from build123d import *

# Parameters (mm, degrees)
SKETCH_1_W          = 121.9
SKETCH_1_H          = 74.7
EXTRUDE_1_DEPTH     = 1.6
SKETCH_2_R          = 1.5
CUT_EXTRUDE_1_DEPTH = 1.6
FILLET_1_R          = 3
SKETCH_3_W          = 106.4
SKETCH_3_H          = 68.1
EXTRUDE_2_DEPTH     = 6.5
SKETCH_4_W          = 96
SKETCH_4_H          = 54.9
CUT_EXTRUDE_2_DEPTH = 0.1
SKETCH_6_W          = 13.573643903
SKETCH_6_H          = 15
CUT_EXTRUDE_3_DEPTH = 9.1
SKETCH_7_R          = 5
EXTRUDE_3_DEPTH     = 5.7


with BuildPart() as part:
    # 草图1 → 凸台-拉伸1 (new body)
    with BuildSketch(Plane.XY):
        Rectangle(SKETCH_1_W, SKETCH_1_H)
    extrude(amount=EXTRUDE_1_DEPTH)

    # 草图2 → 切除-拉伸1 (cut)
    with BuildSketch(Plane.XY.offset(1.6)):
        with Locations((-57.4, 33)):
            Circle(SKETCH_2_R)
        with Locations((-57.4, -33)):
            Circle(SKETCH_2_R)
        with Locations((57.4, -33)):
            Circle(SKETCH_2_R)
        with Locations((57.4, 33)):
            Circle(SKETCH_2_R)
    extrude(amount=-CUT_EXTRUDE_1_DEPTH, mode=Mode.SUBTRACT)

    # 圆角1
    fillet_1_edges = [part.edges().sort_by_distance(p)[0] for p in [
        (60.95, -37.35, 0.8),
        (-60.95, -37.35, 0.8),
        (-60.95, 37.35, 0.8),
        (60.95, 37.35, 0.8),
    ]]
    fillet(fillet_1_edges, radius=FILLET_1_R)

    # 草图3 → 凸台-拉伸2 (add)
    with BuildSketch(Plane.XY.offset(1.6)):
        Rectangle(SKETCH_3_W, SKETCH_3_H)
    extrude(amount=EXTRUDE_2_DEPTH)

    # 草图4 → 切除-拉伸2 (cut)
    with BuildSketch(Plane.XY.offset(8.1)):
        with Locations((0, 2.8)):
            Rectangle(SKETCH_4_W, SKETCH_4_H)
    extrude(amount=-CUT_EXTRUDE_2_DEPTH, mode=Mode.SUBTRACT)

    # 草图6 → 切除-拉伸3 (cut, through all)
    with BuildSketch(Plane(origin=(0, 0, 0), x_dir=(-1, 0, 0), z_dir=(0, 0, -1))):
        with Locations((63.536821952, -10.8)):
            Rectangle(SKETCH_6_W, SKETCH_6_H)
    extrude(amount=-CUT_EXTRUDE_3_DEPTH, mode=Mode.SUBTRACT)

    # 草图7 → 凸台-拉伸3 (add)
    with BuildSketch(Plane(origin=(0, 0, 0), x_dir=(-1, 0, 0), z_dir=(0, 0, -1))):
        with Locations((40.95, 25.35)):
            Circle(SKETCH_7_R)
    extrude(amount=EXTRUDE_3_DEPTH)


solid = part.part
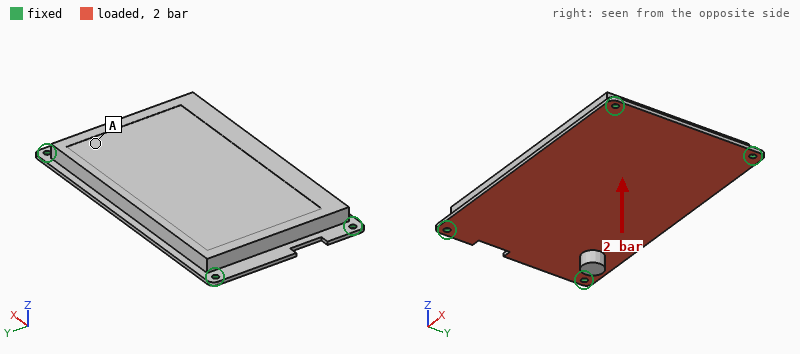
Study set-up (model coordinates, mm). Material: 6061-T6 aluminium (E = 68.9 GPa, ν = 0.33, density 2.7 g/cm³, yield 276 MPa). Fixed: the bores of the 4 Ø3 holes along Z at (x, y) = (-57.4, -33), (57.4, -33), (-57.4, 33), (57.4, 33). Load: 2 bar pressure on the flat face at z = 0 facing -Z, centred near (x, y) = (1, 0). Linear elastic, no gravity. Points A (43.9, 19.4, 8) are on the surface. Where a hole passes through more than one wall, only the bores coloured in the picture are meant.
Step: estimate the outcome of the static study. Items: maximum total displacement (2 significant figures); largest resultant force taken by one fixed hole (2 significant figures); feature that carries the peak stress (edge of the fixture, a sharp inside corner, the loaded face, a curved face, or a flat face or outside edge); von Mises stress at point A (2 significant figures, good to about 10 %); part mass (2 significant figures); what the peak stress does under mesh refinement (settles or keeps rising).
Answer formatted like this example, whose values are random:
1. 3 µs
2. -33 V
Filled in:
1. 0.12 mm
2. 1.0 kN
3. edge of the fixture
4. 15 MPa
5. 170 g
6. keeps rising
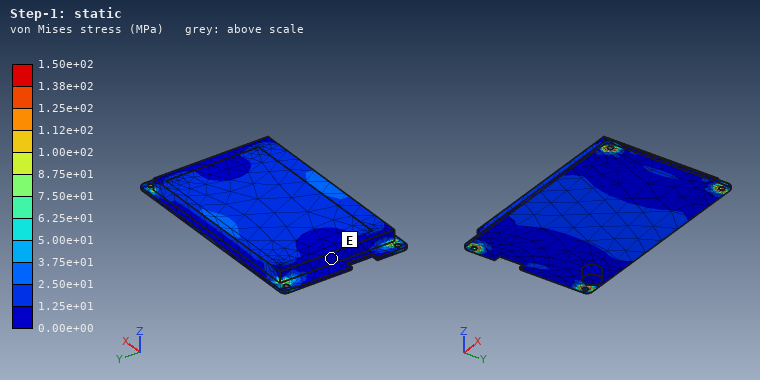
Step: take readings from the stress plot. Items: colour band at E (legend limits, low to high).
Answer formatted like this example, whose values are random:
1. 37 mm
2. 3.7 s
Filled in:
1. 0.00e+00 to 1.25e+01 MPa
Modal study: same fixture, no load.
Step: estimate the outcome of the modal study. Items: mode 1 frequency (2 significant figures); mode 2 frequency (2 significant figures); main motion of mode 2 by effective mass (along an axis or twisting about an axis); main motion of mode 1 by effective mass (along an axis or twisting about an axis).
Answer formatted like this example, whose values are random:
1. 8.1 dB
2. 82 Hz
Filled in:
1. 1600 Hz
2. 3100 Hz
3. twisting about X
4. along Z
